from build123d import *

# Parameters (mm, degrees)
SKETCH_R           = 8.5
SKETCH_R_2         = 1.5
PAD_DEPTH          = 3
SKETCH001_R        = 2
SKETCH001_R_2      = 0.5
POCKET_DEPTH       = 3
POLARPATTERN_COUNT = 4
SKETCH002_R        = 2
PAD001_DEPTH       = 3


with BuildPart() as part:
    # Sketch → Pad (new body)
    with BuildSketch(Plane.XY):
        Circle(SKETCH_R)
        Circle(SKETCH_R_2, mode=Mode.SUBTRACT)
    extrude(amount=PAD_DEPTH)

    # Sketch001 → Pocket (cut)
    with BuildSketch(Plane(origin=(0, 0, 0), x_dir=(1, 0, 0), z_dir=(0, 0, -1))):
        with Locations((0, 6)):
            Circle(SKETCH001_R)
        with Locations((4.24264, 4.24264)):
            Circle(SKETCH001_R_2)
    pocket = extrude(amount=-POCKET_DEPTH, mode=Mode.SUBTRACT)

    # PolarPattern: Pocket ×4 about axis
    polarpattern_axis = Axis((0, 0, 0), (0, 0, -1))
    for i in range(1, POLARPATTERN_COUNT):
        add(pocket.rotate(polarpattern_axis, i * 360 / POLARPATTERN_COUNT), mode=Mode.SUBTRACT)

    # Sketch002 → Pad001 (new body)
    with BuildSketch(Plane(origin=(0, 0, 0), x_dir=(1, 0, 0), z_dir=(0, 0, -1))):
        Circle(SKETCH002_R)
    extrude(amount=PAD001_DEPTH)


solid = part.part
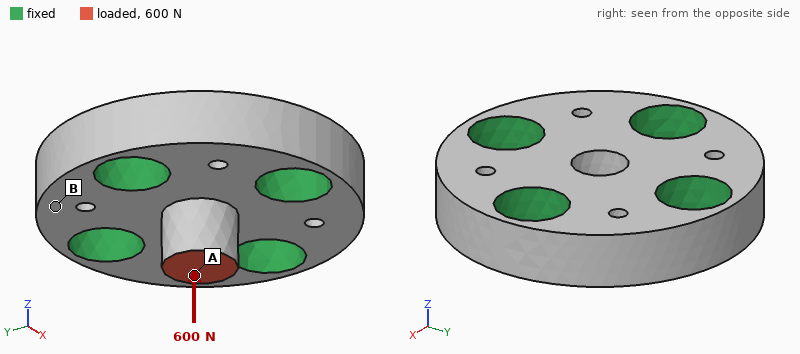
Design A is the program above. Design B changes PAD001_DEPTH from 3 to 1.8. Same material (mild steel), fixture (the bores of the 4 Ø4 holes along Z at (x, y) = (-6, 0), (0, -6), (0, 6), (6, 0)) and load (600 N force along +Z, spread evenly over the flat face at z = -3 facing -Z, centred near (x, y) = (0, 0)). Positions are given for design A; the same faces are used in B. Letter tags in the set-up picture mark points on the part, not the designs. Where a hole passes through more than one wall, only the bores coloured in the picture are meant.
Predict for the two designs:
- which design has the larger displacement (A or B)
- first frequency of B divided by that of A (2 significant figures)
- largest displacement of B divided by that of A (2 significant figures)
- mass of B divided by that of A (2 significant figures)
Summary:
A
1.4
0.88
0.97
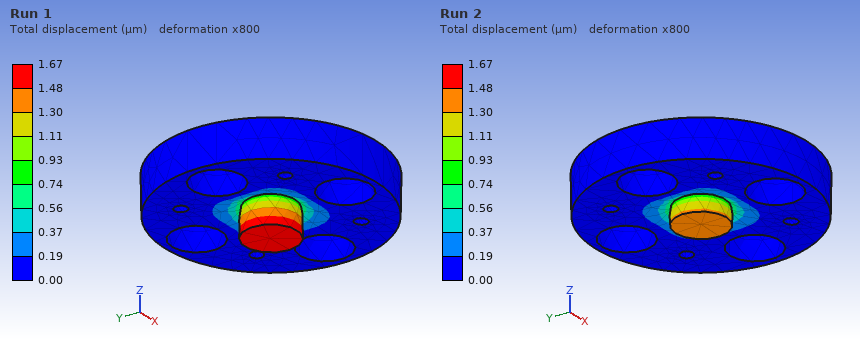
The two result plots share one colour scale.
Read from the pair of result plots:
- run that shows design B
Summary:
Run 2
